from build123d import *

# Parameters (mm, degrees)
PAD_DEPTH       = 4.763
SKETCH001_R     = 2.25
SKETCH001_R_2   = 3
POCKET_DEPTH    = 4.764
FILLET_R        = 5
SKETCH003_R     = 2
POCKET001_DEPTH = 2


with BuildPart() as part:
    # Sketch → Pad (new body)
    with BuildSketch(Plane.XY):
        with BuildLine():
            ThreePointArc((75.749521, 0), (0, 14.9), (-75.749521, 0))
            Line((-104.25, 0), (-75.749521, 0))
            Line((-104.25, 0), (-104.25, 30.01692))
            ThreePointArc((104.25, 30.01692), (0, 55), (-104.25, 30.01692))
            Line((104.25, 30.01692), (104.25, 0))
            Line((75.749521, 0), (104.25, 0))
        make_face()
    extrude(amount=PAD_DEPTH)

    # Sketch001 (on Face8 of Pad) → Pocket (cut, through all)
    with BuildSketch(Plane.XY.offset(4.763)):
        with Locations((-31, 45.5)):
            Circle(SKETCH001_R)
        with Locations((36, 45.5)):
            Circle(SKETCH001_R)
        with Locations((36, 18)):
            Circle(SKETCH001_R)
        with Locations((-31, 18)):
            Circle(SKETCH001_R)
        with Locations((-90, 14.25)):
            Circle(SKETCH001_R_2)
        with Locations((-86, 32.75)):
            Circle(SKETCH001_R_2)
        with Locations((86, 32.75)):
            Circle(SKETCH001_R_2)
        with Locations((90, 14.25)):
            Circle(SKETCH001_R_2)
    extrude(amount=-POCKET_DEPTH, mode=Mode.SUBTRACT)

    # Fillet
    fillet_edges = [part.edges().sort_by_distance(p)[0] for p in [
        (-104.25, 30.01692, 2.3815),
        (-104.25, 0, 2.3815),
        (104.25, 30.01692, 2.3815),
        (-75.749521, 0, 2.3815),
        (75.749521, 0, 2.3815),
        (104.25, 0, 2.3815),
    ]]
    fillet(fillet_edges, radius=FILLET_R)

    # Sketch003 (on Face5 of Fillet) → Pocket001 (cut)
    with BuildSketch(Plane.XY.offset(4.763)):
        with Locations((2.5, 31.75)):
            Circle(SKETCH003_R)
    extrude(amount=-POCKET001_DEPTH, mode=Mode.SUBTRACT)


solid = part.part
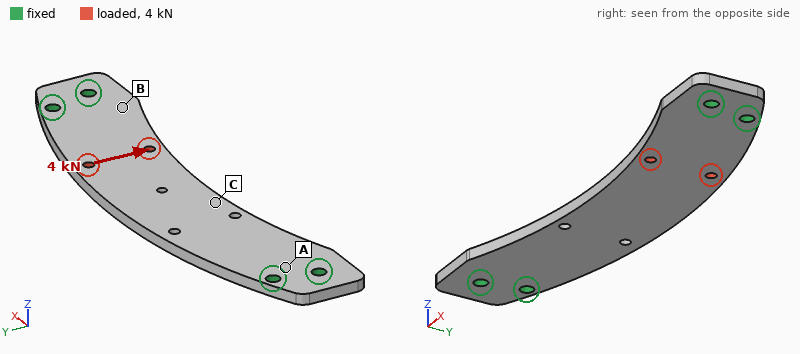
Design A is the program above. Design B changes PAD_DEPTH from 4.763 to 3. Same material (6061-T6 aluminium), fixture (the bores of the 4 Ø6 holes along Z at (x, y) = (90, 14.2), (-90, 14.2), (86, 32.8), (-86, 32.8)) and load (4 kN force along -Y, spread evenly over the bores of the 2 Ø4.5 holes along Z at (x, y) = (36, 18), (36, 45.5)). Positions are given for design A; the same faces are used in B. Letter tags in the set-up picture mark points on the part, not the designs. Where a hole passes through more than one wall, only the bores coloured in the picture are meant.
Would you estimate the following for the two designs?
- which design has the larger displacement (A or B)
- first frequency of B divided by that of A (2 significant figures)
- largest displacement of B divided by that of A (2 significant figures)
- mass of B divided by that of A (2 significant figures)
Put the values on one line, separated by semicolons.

B; 0.64; 1.6; 0.63
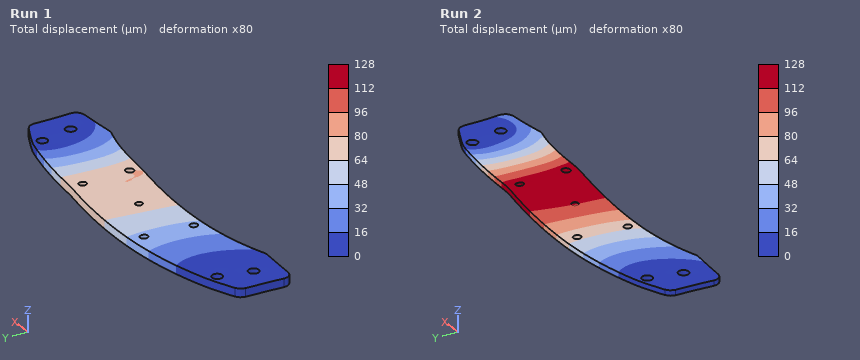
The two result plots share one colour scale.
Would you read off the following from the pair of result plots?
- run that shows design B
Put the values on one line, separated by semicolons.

Run 2
